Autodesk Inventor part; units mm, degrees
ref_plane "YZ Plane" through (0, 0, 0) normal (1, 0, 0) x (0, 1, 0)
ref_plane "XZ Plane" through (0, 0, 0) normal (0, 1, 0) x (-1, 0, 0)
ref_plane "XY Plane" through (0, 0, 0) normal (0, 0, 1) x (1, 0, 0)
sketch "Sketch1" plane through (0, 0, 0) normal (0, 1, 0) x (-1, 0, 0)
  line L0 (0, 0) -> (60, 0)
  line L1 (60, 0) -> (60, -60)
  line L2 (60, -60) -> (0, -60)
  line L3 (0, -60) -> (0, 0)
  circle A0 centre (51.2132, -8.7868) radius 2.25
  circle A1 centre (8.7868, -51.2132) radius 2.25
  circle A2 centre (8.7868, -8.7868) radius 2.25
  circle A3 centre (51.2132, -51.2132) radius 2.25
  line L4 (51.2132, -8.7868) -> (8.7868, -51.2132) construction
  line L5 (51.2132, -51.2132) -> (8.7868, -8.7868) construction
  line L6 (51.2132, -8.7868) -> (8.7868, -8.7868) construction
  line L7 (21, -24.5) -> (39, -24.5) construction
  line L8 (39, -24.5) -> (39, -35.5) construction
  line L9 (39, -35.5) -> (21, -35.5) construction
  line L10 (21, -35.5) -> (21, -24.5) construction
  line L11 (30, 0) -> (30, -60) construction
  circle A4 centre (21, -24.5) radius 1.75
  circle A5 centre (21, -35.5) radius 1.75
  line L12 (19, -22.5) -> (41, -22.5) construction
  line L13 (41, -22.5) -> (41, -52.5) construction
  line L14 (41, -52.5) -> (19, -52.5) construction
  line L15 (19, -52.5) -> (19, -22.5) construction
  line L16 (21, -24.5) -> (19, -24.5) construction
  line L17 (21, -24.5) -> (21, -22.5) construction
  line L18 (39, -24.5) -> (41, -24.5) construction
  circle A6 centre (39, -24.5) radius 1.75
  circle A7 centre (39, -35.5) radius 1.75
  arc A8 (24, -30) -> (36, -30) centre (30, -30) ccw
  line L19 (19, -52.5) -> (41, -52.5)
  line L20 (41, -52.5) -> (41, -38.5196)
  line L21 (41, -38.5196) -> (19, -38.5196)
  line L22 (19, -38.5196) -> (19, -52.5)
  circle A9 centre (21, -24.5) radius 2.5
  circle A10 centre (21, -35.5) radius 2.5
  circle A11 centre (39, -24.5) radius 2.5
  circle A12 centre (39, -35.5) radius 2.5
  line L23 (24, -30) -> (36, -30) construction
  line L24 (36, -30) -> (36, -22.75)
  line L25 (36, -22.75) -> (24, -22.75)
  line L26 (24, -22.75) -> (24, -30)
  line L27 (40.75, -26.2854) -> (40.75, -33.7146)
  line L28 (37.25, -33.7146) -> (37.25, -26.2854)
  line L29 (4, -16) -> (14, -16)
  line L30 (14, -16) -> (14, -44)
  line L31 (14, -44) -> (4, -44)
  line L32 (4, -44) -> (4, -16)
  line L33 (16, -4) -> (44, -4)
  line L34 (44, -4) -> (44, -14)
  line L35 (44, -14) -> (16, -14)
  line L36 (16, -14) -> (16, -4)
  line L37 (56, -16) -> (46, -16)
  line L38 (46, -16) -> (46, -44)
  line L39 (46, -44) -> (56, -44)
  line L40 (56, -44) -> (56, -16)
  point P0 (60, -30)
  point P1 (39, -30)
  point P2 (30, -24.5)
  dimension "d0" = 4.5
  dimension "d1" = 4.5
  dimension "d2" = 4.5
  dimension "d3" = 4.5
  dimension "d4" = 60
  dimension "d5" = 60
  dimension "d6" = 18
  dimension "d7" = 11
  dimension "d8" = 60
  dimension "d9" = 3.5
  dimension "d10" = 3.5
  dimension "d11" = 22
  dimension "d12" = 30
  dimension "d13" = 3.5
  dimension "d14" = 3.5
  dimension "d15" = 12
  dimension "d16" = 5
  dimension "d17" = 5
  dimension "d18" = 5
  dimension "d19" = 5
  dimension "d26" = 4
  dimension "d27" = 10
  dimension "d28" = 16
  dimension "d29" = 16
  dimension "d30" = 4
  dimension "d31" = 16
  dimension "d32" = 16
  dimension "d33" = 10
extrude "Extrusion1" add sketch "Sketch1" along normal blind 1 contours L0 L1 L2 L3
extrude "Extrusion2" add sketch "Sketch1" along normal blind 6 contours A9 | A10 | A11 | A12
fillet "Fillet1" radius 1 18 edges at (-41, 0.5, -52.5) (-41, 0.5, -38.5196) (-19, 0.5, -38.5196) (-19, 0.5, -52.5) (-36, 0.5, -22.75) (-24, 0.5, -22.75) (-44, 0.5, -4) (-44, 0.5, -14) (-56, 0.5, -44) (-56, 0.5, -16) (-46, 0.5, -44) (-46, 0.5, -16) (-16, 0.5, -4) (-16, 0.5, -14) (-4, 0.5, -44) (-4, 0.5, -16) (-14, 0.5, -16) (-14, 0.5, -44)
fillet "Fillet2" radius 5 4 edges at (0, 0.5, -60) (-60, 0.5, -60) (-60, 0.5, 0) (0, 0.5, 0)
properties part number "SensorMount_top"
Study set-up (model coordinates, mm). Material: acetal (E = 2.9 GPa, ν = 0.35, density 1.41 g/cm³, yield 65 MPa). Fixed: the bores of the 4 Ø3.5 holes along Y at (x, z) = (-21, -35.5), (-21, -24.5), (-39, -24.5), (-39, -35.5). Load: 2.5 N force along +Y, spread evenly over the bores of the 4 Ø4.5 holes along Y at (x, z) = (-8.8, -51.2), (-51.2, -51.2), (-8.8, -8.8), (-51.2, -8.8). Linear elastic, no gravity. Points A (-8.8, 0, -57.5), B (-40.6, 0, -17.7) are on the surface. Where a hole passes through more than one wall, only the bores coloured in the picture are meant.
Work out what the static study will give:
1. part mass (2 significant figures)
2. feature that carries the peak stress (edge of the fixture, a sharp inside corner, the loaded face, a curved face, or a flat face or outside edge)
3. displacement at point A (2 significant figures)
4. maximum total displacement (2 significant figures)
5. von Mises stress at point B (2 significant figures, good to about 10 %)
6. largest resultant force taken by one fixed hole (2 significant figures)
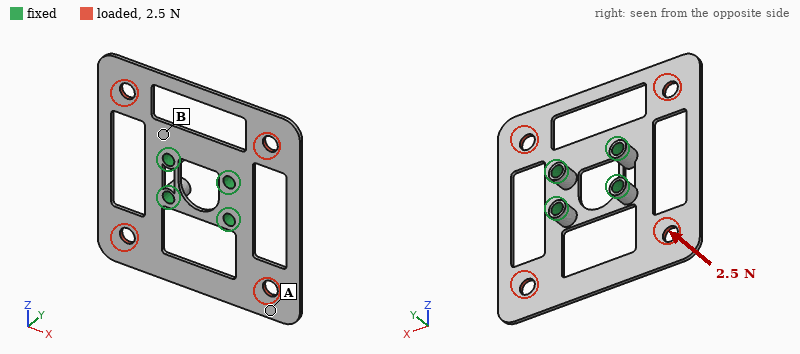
3.3 g
a curved face
0.81 mm
1.0 mm
3.3 MPa
0.76 N
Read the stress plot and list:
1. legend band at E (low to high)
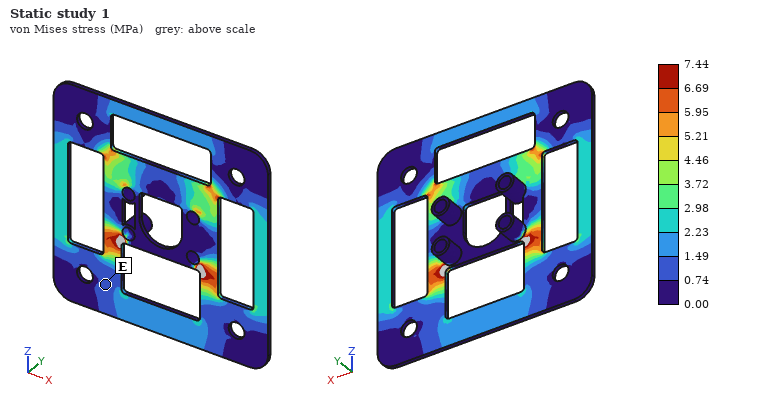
0.74 to 1.49 MPa
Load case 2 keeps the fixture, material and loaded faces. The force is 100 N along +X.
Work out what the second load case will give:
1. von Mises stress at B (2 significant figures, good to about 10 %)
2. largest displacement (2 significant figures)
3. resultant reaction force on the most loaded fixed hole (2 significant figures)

3.9 MPa
0.20 mm
35 N
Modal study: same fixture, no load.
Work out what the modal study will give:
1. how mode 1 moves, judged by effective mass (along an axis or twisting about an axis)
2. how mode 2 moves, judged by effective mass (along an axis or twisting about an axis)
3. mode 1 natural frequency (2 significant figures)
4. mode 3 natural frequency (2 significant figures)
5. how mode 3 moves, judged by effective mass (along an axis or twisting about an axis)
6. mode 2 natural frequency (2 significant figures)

along Y
twisting about Z
200 Hz
250 Hz
along Y
240 Hz
